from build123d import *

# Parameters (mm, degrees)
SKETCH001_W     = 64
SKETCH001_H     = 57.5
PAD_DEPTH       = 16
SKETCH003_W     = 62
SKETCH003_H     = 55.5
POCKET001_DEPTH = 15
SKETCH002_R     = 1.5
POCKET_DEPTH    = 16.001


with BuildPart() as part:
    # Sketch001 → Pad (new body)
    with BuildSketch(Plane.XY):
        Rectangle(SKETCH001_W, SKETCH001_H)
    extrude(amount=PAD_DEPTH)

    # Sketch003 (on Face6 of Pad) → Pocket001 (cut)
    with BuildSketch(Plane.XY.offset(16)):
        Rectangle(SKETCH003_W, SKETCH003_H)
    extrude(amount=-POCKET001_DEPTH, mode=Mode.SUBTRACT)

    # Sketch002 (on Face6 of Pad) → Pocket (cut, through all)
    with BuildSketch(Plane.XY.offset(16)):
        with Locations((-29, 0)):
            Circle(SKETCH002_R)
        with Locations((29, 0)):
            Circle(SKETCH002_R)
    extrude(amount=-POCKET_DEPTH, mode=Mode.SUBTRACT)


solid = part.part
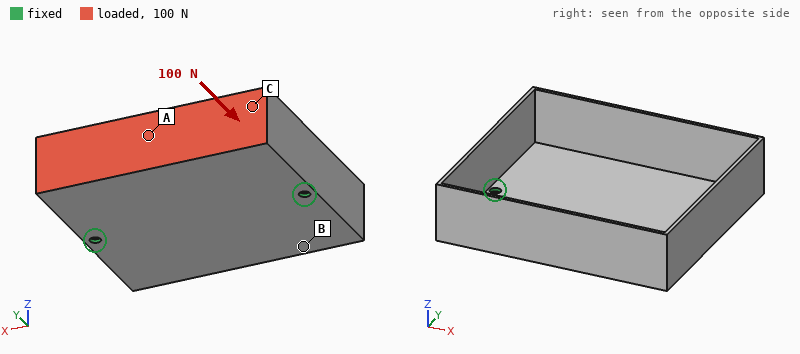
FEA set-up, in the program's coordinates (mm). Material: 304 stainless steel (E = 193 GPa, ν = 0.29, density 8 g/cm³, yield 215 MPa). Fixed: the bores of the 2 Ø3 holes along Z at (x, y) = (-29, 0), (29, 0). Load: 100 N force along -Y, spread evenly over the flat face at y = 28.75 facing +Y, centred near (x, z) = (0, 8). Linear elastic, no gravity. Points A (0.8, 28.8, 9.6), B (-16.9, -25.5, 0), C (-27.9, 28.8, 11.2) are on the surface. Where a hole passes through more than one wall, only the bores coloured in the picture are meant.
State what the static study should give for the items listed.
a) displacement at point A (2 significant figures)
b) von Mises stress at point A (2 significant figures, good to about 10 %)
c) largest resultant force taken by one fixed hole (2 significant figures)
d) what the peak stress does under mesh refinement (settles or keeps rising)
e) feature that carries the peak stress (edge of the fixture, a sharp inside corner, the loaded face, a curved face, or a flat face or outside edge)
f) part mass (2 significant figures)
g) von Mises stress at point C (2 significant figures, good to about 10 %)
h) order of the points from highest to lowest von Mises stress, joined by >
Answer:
62 µm
9.4 MPa
51 N
keeps rising
edge of the fixture
58 g
31 MPa
C > A > B
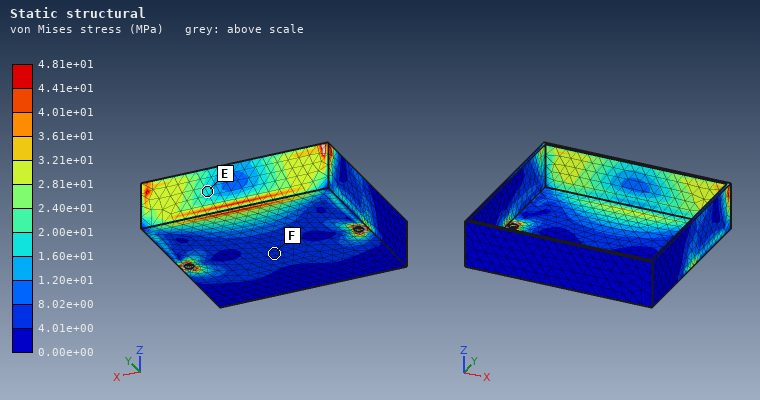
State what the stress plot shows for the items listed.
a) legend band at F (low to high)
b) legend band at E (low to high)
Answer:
4.01e+00 to 8.02e+00 MPa
1.60e+01 to 2.00e+01 MPa
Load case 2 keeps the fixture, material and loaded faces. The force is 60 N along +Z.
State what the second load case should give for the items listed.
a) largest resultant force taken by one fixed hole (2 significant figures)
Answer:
31 N
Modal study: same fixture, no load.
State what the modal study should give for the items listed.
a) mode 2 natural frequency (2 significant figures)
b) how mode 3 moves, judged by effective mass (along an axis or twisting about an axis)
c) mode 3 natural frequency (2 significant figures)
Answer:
1200 Hz
along Z
1900 Hz
